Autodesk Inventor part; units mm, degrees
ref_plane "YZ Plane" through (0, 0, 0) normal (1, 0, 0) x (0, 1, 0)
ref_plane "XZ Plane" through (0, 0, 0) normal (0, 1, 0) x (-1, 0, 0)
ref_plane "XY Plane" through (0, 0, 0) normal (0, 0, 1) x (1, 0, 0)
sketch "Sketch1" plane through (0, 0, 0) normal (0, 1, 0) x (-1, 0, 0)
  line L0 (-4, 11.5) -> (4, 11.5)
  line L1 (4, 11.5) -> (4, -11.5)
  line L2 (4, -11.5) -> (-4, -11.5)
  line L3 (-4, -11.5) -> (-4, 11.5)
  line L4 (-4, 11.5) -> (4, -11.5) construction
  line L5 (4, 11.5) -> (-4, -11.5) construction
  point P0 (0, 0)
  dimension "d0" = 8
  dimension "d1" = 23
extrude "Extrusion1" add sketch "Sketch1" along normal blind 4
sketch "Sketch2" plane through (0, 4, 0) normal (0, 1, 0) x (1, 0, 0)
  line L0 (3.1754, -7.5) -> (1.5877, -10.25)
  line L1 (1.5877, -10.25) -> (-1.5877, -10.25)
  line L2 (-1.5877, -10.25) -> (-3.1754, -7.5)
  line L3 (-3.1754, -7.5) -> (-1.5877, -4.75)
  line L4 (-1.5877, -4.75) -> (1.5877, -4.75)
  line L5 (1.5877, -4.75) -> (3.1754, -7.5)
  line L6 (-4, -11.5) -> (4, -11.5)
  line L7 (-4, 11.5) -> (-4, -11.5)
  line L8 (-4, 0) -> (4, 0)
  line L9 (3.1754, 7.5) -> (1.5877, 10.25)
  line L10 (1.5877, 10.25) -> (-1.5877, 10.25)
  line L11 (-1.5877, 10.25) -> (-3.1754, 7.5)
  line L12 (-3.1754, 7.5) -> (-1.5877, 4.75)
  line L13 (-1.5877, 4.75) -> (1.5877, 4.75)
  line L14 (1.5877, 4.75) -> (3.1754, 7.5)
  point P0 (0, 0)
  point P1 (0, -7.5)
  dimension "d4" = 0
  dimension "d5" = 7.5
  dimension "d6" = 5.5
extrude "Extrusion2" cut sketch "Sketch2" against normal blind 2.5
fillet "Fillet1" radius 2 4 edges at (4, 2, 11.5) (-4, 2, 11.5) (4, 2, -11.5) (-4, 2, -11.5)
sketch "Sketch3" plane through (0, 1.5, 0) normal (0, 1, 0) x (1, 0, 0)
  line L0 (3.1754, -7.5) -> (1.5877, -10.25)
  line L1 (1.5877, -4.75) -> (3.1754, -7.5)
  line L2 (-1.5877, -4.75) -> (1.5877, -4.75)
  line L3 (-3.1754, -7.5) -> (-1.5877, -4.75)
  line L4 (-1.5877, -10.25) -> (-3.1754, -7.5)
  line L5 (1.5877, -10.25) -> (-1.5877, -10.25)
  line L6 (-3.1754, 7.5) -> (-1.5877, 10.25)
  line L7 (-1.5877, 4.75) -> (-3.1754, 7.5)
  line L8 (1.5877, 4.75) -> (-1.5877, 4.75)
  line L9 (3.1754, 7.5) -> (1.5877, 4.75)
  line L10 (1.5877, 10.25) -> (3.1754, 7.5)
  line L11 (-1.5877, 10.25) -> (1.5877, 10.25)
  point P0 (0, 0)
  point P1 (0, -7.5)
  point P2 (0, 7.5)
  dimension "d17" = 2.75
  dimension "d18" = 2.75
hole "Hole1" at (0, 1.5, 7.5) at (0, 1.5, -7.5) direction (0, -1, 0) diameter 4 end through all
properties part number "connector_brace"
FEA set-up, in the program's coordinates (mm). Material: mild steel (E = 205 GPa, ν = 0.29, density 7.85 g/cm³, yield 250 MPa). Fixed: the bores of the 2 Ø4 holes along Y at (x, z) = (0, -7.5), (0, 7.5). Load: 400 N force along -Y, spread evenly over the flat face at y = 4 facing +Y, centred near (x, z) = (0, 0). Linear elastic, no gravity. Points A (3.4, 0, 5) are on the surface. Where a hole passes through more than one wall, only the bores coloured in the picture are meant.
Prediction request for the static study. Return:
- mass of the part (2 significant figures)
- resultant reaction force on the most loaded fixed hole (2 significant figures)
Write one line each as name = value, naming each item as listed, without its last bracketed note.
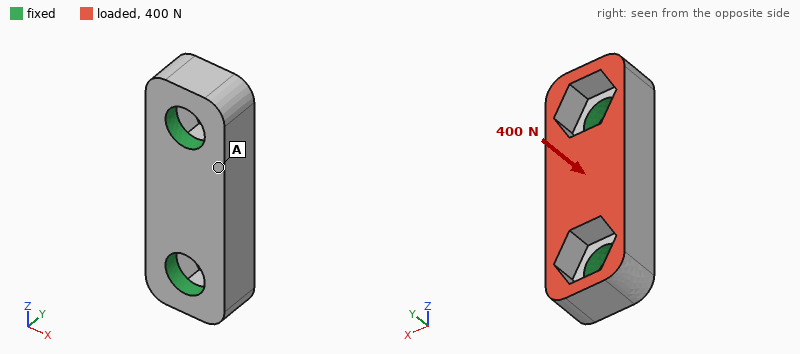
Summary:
mass of the part = 4.3 g
resultant reaction force on the most loaded fixed hole = 210 N
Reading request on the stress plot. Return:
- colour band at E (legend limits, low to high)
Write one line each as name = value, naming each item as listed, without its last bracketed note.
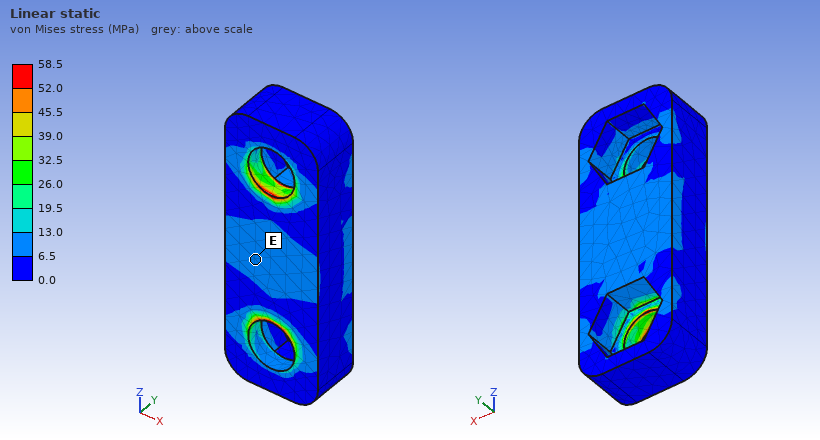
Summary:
colour band at E = 6.5 to 13.0 MPa
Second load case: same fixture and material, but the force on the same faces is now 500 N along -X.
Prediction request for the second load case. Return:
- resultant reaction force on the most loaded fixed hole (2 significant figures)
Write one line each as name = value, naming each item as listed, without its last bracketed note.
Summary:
resultant reaction force on the most loaded fixed hole = 250 N
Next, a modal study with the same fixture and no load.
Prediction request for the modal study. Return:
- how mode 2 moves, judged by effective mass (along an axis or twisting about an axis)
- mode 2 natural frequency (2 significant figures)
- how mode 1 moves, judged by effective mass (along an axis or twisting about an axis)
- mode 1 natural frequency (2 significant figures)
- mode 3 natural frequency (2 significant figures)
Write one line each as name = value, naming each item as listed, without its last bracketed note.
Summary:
how mode 2 moves, judged by effective mass = along Y
mode 2 natural frequency = 62 kHz
how mode 1 moves, judged by effective mass = along X
mode 1 natural frequency = 49 kHz
mode 3 natural frequency = 85 kHz
